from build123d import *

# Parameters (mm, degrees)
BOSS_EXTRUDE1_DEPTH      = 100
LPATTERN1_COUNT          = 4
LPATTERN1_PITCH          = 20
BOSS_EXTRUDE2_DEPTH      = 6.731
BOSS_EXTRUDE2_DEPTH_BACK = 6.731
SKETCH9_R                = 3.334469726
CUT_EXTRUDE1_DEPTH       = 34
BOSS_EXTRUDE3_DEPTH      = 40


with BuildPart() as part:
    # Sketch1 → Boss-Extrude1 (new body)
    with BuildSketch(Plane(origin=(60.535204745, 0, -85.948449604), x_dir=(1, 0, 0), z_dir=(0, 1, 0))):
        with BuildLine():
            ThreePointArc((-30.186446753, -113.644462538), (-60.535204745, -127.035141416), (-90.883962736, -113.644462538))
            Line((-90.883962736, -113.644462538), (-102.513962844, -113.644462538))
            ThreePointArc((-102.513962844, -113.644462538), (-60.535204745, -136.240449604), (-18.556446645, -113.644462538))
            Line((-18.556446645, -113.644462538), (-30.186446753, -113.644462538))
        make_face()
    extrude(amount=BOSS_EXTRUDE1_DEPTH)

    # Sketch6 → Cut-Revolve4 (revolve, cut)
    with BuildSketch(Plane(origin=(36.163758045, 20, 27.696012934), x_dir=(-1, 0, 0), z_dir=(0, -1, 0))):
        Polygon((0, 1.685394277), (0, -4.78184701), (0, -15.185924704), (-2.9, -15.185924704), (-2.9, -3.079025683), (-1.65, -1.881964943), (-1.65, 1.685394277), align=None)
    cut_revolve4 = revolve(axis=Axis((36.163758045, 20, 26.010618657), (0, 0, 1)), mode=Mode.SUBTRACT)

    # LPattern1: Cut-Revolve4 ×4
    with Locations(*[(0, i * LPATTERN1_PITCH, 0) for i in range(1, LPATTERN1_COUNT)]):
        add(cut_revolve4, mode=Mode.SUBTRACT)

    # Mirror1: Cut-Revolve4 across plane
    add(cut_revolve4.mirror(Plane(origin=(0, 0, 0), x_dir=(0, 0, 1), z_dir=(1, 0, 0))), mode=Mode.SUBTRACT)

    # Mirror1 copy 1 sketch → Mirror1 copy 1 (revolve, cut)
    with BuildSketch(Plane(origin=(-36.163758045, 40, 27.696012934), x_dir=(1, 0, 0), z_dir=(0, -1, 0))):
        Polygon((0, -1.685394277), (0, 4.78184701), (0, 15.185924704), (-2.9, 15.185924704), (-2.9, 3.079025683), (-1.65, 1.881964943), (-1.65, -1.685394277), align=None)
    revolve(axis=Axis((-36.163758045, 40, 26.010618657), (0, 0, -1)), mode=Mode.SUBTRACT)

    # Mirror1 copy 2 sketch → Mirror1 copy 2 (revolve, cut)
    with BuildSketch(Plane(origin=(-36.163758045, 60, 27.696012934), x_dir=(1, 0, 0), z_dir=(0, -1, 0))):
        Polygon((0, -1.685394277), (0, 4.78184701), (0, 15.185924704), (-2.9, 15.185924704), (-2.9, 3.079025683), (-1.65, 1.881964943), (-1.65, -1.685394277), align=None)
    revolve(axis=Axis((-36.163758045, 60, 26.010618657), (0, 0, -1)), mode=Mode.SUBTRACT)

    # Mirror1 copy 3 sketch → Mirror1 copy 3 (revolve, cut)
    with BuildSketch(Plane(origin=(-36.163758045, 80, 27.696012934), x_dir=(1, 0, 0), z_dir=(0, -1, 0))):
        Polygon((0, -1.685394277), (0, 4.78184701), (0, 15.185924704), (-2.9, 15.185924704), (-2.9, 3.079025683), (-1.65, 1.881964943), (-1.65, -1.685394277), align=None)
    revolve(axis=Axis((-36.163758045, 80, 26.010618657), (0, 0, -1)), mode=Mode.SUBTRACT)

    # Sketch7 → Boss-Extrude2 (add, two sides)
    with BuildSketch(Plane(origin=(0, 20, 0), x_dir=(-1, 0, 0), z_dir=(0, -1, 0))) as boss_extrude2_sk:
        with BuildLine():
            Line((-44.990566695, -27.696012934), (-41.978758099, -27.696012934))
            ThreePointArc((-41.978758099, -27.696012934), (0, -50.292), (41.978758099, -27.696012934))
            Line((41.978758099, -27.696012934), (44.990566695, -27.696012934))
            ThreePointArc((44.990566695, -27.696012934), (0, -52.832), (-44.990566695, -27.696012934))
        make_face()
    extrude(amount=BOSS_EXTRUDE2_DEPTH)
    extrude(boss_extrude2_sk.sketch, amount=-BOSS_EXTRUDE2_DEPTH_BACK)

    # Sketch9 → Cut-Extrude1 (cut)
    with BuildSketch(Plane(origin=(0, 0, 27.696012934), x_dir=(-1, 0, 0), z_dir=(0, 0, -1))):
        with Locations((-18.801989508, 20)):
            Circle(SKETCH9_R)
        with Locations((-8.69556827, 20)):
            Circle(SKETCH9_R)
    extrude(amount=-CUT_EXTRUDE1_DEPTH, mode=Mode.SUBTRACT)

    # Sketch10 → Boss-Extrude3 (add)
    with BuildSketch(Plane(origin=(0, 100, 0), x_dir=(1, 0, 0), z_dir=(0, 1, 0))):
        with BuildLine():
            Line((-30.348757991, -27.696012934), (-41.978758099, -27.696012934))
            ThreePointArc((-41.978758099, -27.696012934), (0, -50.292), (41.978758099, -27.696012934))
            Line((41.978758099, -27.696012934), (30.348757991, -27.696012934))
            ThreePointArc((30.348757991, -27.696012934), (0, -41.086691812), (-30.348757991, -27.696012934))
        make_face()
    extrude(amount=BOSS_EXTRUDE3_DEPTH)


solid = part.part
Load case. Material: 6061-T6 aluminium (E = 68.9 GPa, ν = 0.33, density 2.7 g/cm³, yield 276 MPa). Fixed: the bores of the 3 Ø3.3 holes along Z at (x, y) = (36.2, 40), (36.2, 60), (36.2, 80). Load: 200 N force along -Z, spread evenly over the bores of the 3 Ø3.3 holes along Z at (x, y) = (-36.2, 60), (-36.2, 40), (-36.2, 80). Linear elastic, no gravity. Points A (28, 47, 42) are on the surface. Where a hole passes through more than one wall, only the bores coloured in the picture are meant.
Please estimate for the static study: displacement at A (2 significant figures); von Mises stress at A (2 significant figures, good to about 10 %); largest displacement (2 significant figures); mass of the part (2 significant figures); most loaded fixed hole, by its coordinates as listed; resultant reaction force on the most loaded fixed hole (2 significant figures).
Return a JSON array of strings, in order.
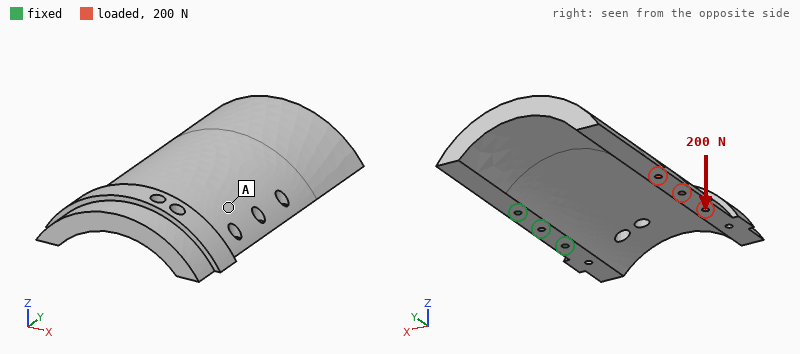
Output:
["0.074 mm", "10 MPa", "0.46 mm", "300 g", "(36.2, 60)", "130 N"]
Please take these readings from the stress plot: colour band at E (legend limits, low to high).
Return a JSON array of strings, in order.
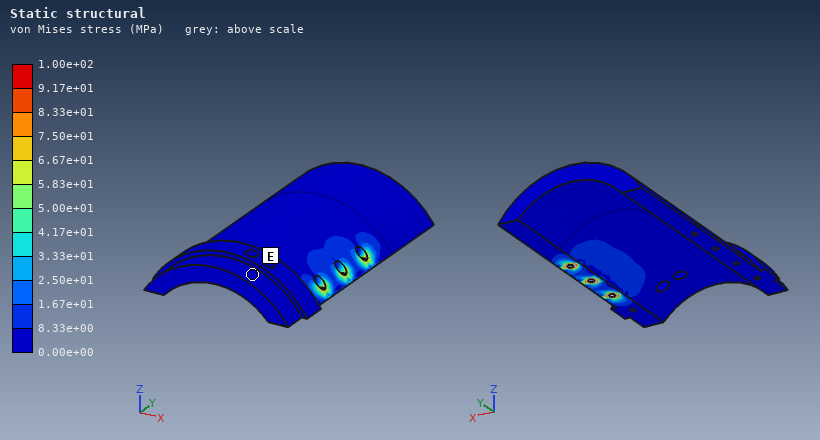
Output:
["0.00e+00 to 8.33e+00 MPa"]
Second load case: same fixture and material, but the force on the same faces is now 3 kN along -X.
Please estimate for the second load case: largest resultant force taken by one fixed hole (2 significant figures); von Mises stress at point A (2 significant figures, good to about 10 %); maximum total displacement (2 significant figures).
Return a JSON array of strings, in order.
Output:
["1.2 kN", "15 MPa", "0.27 mm"]
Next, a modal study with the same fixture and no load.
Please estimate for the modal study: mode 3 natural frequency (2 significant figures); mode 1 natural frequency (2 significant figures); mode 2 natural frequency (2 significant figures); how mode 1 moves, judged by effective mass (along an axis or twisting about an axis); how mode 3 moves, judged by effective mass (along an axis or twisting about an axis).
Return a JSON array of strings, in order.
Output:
["1900 Hz", "340 Hz", "790 Hz", "along Z", "along Y"]
